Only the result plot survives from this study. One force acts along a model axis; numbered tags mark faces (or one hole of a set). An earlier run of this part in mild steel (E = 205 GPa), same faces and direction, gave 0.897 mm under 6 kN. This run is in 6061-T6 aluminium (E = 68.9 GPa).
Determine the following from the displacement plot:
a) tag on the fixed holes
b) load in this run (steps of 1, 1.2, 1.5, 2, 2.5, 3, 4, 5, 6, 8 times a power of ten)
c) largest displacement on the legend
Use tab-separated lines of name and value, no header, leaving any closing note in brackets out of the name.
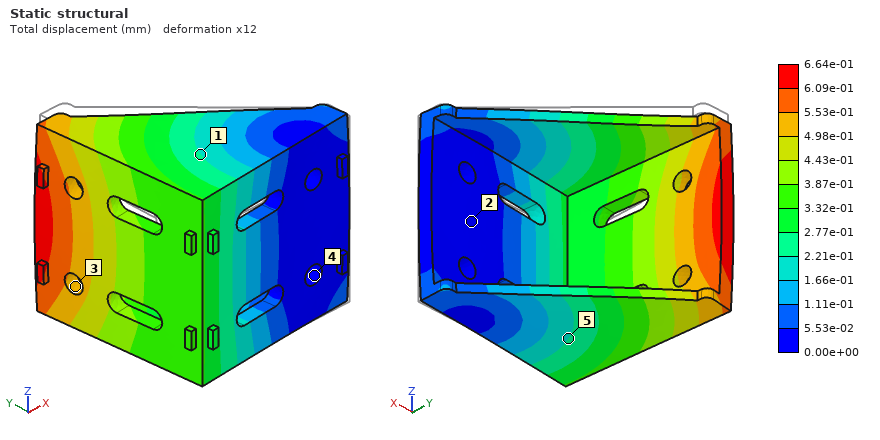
tag on the fixed holes	4
load in this run	1.5 kN
largest displacement on the legend	6.64e-01 mm
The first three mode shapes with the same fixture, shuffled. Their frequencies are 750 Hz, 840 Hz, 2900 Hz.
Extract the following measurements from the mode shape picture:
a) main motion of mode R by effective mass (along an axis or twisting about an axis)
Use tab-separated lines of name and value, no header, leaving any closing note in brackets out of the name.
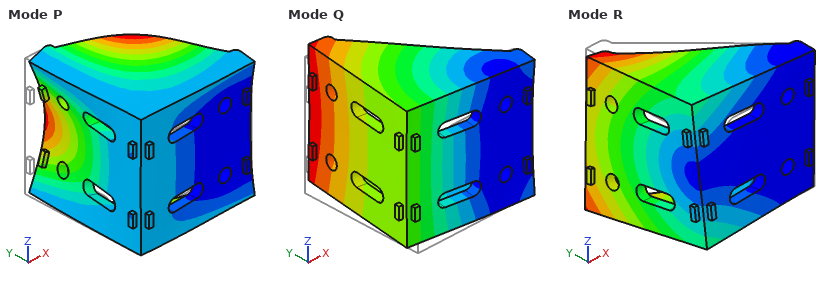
main motion of mode R by effective mass	along Z
